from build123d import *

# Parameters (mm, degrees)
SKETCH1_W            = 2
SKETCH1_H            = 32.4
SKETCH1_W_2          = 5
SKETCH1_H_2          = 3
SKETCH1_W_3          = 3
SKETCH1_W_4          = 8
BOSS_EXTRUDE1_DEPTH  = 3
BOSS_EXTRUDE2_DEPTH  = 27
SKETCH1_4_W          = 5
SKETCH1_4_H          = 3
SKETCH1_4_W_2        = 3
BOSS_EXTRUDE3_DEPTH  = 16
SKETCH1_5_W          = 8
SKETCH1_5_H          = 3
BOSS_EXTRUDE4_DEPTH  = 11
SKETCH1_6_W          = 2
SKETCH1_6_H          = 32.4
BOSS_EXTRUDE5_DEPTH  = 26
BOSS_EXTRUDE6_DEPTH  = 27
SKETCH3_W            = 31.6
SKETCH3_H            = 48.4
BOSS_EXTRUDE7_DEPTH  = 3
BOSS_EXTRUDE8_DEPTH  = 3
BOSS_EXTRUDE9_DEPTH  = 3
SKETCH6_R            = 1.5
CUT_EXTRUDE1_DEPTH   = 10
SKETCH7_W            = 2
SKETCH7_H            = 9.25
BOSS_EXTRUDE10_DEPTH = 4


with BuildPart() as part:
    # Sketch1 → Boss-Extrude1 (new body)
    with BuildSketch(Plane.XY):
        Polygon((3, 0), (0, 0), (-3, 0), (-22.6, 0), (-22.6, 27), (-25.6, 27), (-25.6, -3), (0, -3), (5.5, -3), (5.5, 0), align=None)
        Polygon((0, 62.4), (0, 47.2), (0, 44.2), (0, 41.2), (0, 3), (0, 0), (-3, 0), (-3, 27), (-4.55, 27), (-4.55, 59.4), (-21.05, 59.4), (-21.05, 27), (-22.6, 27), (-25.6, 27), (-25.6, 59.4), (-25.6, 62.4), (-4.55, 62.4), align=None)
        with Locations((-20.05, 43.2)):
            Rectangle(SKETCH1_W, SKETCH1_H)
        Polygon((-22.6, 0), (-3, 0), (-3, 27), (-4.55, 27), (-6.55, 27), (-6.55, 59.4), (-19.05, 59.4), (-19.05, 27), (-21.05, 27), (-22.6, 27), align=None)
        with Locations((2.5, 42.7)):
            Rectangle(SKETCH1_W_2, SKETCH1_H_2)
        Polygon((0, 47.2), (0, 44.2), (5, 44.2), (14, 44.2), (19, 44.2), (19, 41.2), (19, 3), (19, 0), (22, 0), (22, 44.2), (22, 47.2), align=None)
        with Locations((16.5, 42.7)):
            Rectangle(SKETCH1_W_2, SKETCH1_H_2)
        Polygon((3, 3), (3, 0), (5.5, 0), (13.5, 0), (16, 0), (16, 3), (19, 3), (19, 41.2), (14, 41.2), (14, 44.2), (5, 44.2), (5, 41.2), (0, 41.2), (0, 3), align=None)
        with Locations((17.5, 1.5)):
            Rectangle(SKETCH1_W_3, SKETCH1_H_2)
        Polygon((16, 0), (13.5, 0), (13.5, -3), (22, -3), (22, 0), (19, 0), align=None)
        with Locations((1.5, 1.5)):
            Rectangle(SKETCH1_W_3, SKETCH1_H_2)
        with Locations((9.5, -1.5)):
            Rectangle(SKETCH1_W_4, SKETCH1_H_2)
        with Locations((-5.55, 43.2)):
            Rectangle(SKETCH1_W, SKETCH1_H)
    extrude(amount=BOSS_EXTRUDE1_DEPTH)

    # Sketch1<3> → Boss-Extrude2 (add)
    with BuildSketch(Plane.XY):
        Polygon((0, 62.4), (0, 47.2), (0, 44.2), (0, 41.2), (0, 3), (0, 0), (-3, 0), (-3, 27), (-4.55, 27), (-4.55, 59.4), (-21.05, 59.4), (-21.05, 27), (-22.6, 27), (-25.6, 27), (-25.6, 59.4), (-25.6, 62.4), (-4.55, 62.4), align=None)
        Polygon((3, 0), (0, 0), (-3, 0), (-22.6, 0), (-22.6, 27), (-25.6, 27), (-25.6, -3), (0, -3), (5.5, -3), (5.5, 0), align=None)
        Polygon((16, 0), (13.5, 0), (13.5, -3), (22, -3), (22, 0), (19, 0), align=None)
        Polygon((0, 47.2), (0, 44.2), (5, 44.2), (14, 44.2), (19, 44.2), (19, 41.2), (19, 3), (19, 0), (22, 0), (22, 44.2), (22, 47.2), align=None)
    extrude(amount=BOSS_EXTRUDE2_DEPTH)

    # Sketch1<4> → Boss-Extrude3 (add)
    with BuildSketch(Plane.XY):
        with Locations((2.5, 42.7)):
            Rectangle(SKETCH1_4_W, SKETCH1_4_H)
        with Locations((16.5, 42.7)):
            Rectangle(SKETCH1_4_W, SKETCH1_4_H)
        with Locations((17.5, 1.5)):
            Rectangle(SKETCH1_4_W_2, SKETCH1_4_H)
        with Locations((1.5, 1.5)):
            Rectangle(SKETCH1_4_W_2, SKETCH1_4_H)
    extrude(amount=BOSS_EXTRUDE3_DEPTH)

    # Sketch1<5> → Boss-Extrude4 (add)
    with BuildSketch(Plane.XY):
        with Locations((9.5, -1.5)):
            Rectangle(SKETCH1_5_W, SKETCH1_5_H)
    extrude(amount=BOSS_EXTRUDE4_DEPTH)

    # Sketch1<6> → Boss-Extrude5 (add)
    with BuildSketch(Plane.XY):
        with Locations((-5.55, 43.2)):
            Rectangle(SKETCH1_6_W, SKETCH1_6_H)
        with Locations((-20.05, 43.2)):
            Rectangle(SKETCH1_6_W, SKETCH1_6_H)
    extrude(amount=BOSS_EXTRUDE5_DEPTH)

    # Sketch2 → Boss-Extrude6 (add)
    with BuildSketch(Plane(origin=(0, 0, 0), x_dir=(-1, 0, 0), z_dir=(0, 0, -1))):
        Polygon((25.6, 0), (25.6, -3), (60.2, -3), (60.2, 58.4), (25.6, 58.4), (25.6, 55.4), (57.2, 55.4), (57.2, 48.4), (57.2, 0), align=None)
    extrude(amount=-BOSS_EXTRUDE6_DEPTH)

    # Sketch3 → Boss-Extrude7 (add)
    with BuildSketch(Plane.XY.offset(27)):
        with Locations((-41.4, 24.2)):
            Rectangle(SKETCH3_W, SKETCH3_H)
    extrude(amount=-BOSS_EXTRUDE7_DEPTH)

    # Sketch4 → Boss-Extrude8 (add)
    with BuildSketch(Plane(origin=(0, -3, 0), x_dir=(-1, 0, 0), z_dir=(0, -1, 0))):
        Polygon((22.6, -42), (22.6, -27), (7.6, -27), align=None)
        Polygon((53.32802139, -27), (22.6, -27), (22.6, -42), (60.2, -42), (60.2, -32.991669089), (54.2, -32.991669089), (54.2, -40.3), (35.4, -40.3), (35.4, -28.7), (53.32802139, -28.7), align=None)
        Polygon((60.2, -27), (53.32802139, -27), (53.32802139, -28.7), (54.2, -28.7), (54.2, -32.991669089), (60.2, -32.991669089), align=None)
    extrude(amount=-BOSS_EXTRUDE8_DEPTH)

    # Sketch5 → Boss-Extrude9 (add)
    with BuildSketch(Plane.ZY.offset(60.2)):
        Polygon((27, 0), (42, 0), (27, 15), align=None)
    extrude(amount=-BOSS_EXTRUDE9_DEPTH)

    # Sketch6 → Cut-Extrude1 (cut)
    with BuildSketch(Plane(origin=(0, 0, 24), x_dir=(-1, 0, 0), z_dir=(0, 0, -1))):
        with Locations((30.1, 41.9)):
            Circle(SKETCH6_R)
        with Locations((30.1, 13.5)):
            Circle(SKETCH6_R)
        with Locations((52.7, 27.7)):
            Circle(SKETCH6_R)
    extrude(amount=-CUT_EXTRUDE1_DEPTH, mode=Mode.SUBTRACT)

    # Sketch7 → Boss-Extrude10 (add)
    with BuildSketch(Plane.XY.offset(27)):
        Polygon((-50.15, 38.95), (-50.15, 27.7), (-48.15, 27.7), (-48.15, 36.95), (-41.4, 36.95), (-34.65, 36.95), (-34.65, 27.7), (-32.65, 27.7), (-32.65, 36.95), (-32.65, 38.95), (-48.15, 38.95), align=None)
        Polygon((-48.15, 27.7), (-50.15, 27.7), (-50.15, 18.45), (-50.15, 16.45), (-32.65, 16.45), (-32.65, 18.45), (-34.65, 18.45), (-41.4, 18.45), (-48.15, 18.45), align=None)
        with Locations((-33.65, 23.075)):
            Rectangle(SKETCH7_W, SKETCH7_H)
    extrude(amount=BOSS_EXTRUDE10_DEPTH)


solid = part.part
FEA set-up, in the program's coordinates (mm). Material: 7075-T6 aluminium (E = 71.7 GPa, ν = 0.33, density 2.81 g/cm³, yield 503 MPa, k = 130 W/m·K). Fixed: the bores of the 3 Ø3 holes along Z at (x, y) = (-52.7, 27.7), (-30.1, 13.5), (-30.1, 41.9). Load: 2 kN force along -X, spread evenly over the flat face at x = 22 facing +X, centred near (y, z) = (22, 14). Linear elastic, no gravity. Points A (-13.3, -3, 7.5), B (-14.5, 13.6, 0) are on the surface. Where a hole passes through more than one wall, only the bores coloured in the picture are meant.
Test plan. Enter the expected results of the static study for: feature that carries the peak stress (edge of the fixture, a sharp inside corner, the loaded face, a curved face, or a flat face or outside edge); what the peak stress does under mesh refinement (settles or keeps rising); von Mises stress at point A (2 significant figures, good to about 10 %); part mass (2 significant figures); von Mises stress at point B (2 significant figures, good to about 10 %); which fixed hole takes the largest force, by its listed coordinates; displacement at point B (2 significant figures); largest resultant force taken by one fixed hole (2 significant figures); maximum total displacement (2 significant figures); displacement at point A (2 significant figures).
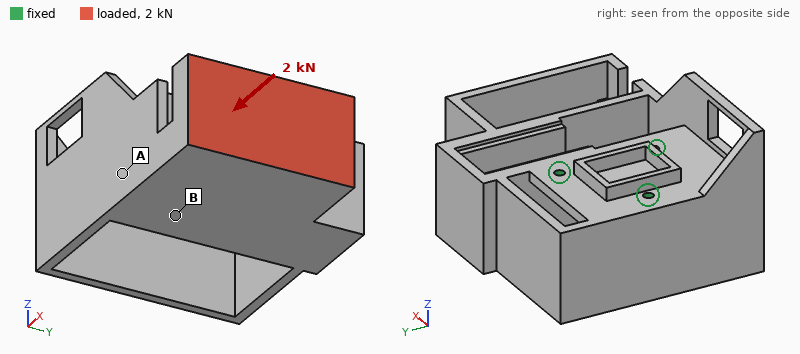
edge of the fixture
keeps rising
15 MPa
140 g
8.2 MPa
(-30.1, 13.5)
0.081 mm
1.1 kN
0.25 mm
0.073 mm
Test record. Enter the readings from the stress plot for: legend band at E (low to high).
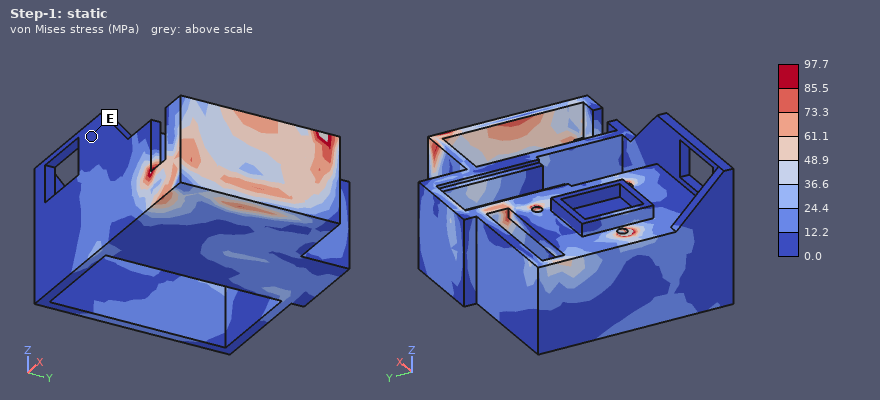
0.0 to 12.2 MPa
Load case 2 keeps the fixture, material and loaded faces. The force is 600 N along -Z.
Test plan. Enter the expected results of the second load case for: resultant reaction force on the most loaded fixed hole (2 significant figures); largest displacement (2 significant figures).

1.0 kN
0.20 mm
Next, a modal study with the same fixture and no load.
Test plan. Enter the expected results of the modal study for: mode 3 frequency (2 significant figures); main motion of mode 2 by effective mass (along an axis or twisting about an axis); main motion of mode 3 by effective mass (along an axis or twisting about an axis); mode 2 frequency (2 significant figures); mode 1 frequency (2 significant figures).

2700 Hz
along Y
along Y
1800 Hz
1600 Hz
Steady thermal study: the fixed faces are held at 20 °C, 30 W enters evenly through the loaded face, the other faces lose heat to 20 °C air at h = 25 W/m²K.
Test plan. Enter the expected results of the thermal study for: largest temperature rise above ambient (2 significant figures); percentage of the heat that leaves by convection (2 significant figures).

52 K
39 %
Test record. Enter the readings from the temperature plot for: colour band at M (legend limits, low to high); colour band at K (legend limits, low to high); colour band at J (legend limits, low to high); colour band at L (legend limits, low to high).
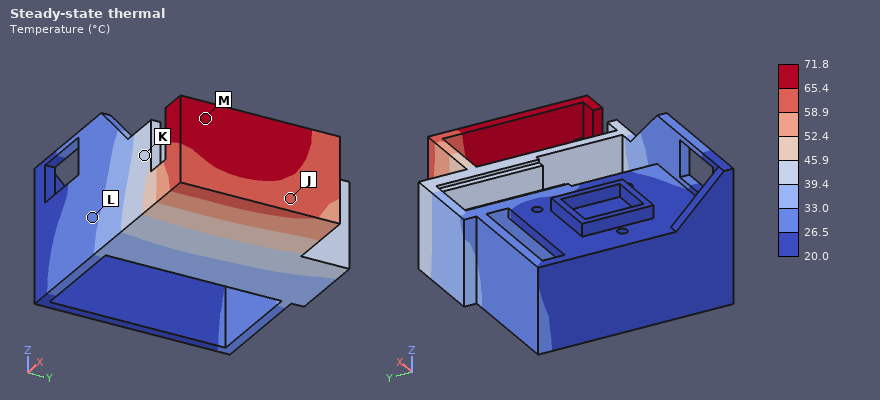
65.4 to 71.8 °C
39.4 to 45.9 °C
58.9 to 65.4 °C
26.5 to 33.0 °C
